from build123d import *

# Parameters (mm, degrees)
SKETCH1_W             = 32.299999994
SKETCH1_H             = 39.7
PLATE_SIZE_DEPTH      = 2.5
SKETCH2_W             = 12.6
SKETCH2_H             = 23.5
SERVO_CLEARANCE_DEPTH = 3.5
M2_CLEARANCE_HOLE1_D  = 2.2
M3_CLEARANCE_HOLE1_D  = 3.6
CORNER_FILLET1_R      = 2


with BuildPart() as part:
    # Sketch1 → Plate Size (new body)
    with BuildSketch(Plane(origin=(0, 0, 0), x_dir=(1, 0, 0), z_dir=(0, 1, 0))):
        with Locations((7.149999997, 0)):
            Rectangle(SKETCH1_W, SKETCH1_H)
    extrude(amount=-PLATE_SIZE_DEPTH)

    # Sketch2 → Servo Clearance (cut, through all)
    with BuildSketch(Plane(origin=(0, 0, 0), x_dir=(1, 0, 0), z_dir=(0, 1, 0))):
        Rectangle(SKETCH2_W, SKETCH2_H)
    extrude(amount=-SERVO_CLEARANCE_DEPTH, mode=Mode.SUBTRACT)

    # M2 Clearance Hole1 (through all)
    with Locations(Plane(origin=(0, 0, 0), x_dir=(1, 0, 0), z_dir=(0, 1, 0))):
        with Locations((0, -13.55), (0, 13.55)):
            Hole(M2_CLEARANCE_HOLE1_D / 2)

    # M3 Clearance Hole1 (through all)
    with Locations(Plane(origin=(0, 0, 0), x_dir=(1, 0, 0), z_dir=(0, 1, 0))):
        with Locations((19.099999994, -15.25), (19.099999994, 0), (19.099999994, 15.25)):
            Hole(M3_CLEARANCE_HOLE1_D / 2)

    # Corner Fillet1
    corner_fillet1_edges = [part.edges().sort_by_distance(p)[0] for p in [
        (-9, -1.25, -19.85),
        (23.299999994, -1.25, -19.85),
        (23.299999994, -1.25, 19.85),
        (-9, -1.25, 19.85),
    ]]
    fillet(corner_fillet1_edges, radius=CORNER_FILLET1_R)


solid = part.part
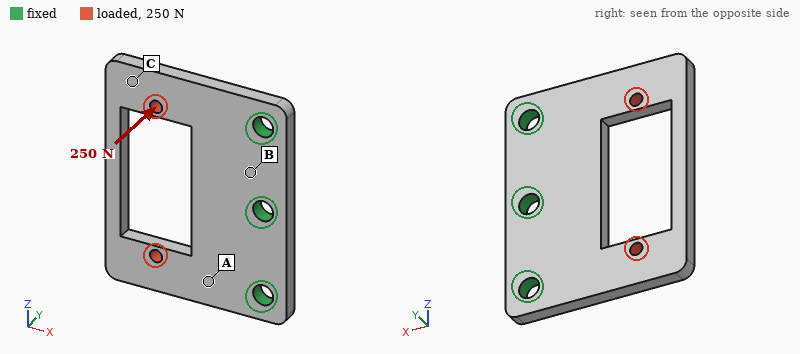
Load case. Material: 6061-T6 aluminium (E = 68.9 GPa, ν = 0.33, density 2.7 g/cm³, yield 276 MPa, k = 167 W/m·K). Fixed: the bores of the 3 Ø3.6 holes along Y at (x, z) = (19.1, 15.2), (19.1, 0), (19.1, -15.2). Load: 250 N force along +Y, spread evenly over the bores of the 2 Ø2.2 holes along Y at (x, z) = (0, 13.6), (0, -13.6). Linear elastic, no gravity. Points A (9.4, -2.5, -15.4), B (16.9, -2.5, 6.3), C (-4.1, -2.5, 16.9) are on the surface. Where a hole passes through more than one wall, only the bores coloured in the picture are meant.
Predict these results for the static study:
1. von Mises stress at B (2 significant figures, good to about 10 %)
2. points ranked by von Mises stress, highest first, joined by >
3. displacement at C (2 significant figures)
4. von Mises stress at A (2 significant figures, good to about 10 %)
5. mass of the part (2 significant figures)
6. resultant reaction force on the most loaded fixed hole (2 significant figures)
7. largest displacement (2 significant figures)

51 MPa
A > B > C
0.27 mm
93 MPa
6.4 g
94 N
0.36 mm
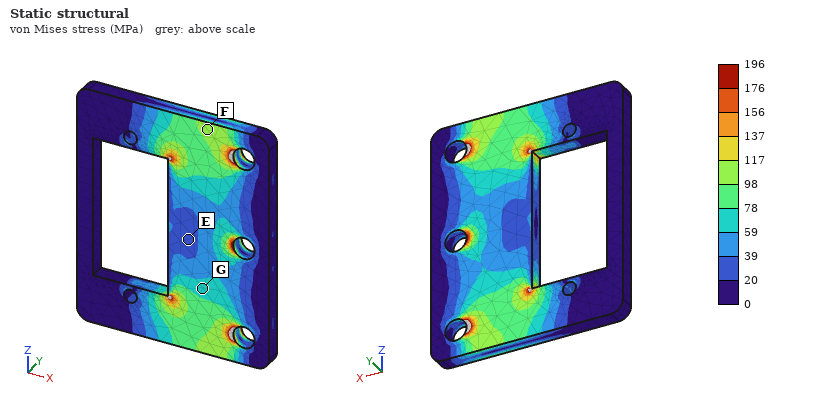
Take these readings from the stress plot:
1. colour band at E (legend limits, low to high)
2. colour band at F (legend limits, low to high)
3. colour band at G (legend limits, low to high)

20 to 39 MPa
98 to 117 MPa
59 to 78 MPa
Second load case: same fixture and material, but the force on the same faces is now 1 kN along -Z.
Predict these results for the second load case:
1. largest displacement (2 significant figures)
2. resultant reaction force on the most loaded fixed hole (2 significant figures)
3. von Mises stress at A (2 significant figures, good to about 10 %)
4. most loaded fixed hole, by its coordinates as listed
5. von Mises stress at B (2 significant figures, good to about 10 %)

76 µm
690 N
21 MPa
(19.1, 0)
26 MPa
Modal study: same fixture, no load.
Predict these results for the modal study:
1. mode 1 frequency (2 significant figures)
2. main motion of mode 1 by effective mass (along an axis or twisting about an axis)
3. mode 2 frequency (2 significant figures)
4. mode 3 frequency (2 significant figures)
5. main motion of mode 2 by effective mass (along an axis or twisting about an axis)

2900 Hz
along Y
4200 Hz
10000 Hz
twisting about X
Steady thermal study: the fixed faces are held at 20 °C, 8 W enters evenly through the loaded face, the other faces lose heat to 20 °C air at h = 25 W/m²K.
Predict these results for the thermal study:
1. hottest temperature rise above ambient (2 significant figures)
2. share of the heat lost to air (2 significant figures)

19 K
5.4 %
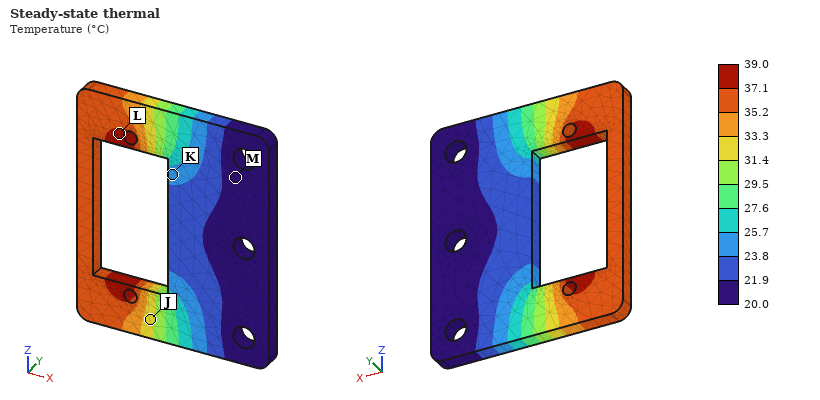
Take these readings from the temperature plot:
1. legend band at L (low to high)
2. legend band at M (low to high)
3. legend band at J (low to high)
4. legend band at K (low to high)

37.1 to 39.0 °C
20.0 to 21.9 °C
31.4 to 33.3 °C
23.8 to 25.7 °C
